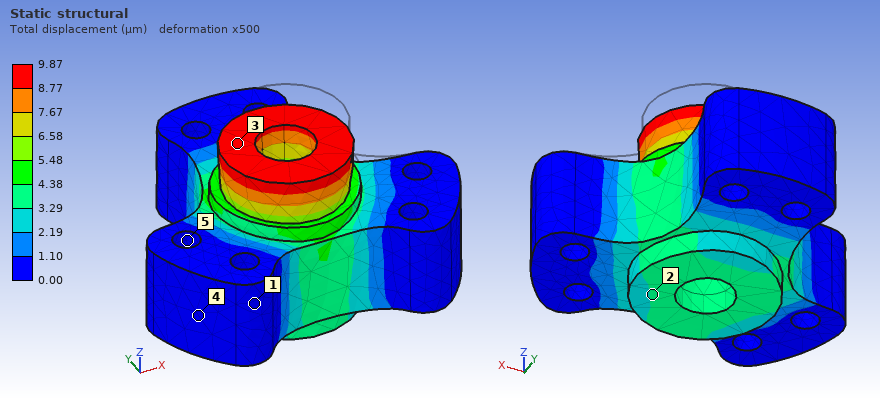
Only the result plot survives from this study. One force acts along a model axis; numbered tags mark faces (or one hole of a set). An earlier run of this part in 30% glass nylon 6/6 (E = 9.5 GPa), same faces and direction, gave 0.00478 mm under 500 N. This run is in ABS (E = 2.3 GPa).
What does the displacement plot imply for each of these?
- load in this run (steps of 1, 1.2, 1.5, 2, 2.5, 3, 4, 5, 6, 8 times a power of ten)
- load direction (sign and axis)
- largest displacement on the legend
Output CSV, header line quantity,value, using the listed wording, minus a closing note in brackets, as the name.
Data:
quantity,value
load in this run,250 N
load direction,-Z
largest displacement on the legend,9.87 µm
